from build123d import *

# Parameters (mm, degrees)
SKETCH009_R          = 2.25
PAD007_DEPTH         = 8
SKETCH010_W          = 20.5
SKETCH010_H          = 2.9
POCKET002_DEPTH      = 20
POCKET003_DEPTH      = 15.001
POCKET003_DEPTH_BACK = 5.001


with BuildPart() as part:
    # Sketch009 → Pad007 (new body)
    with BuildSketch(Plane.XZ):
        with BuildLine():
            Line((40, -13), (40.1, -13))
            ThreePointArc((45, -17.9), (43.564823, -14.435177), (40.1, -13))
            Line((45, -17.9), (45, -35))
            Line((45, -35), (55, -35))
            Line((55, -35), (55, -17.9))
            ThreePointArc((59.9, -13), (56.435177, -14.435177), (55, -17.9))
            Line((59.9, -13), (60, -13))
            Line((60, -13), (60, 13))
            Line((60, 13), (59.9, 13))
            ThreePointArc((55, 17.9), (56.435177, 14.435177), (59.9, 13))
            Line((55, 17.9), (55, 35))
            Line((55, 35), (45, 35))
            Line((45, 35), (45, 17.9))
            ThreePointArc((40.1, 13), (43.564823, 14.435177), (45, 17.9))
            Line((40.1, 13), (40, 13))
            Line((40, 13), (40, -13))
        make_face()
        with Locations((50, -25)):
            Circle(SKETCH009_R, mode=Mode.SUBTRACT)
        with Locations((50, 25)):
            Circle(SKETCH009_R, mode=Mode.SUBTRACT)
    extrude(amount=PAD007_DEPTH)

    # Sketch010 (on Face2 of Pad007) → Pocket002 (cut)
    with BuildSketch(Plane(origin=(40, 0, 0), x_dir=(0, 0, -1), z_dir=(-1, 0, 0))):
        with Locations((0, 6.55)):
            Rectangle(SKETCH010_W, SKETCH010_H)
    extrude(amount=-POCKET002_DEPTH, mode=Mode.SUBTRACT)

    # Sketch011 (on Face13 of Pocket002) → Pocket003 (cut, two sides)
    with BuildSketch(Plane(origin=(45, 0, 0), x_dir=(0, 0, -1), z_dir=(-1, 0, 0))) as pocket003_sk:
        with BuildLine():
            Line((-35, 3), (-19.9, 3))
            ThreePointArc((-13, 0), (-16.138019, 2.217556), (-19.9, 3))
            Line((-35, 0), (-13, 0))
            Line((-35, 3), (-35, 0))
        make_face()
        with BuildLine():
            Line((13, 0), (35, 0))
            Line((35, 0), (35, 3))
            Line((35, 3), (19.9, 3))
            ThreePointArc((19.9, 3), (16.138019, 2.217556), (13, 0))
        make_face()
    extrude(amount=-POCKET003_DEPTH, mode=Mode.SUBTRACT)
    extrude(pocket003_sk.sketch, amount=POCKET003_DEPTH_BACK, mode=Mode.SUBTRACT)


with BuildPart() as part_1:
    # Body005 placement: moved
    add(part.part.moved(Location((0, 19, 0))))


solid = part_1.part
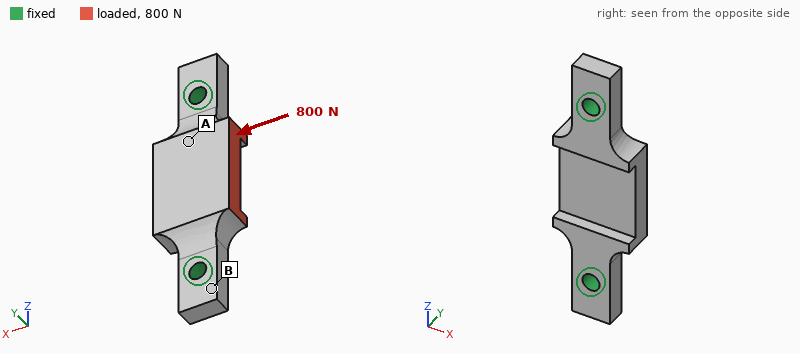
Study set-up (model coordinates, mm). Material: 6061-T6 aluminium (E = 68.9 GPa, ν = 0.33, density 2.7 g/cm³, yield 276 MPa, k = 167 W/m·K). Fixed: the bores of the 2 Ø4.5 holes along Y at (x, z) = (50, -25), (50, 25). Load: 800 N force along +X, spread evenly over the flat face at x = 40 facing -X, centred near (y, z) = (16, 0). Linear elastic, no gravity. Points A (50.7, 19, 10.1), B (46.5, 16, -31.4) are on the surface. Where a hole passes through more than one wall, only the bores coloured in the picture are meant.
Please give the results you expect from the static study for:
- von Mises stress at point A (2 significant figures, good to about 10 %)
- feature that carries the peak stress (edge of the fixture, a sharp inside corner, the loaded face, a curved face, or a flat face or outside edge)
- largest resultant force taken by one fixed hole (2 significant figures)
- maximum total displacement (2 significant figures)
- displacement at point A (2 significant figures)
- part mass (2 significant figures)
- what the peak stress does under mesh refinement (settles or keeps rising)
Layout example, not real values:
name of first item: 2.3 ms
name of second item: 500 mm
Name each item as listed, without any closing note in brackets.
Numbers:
von Mises stress at point A: 11 MPa
feature that carries the peak stress: edge of the fixture
largest resultant force taken by one fixed hole: 400 N
maximum total displacement: 21 µm
displacement at point A: 14 µm
part mass: 14 g
what the peak stress does under mesh refinement: keeps rising
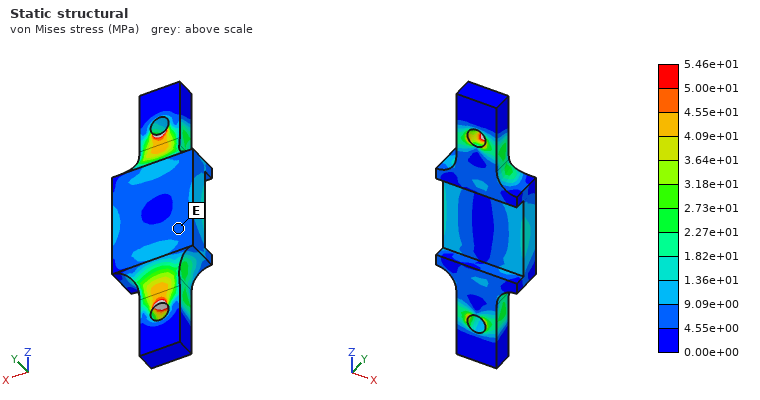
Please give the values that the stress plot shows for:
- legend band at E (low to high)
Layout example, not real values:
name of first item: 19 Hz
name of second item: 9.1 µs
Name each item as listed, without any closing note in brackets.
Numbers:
legend band at E: 4.55e+00 to 9.09e+00 MPa
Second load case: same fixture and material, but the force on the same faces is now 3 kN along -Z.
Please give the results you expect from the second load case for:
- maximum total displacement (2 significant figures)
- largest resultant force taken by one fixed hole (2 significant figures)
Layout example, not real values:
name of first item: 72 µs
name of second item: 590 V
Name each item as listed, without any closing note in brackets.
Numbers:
maximum total displacement: 23 µm
largest resultant force taken by one fixed hole: 1.7 kN
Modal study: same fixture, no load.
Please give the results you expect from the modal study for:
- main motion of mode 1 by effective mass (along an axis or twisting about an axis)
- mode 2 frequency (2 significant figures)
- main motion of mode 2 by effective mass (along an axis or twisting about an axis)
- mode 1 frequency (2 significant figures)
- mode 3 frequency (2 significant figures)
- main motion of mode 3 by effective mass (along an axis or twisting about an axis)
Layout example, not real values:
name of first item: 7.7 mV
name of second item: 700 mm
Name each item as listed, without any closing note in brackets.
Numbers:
main motion of mode 1 by effective mass: along X
mode 2 frequency: 11 kHz
main motion of mode 2 by effective mass: along Y
mode 1 frequency: 10 kHz
mode 3 frequency: 18 kHz
main motion of mode 3 by effective mass: along X
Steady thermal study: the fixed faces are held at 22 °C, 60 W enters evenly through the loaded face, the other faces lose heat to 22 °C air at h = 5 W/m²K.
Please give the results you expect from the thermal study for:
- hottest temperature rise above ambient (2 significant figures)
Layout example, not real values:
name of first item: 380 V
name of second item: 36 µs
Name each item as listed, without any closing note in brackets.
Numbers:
hottest temperature rise above ambient: 62 K
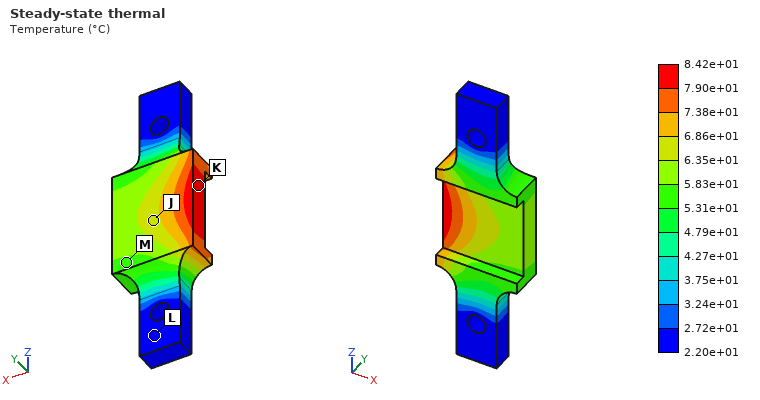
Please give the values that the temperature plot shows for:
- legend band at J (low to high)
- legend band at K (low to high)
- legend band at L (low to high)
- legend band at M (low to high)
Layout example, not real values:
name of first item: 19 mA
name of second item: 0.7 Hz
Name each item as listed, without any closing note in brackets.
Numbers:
legend band at J: 6.35e+01 to 6.86e+01 °C
legend band at K: 7.90e+01 to 8.42e+01 °C
legend band at L: 2.20e+01 to 2.72e+01 °C
legend band at M: 5.31e+01 to 5.83e+01 °C
